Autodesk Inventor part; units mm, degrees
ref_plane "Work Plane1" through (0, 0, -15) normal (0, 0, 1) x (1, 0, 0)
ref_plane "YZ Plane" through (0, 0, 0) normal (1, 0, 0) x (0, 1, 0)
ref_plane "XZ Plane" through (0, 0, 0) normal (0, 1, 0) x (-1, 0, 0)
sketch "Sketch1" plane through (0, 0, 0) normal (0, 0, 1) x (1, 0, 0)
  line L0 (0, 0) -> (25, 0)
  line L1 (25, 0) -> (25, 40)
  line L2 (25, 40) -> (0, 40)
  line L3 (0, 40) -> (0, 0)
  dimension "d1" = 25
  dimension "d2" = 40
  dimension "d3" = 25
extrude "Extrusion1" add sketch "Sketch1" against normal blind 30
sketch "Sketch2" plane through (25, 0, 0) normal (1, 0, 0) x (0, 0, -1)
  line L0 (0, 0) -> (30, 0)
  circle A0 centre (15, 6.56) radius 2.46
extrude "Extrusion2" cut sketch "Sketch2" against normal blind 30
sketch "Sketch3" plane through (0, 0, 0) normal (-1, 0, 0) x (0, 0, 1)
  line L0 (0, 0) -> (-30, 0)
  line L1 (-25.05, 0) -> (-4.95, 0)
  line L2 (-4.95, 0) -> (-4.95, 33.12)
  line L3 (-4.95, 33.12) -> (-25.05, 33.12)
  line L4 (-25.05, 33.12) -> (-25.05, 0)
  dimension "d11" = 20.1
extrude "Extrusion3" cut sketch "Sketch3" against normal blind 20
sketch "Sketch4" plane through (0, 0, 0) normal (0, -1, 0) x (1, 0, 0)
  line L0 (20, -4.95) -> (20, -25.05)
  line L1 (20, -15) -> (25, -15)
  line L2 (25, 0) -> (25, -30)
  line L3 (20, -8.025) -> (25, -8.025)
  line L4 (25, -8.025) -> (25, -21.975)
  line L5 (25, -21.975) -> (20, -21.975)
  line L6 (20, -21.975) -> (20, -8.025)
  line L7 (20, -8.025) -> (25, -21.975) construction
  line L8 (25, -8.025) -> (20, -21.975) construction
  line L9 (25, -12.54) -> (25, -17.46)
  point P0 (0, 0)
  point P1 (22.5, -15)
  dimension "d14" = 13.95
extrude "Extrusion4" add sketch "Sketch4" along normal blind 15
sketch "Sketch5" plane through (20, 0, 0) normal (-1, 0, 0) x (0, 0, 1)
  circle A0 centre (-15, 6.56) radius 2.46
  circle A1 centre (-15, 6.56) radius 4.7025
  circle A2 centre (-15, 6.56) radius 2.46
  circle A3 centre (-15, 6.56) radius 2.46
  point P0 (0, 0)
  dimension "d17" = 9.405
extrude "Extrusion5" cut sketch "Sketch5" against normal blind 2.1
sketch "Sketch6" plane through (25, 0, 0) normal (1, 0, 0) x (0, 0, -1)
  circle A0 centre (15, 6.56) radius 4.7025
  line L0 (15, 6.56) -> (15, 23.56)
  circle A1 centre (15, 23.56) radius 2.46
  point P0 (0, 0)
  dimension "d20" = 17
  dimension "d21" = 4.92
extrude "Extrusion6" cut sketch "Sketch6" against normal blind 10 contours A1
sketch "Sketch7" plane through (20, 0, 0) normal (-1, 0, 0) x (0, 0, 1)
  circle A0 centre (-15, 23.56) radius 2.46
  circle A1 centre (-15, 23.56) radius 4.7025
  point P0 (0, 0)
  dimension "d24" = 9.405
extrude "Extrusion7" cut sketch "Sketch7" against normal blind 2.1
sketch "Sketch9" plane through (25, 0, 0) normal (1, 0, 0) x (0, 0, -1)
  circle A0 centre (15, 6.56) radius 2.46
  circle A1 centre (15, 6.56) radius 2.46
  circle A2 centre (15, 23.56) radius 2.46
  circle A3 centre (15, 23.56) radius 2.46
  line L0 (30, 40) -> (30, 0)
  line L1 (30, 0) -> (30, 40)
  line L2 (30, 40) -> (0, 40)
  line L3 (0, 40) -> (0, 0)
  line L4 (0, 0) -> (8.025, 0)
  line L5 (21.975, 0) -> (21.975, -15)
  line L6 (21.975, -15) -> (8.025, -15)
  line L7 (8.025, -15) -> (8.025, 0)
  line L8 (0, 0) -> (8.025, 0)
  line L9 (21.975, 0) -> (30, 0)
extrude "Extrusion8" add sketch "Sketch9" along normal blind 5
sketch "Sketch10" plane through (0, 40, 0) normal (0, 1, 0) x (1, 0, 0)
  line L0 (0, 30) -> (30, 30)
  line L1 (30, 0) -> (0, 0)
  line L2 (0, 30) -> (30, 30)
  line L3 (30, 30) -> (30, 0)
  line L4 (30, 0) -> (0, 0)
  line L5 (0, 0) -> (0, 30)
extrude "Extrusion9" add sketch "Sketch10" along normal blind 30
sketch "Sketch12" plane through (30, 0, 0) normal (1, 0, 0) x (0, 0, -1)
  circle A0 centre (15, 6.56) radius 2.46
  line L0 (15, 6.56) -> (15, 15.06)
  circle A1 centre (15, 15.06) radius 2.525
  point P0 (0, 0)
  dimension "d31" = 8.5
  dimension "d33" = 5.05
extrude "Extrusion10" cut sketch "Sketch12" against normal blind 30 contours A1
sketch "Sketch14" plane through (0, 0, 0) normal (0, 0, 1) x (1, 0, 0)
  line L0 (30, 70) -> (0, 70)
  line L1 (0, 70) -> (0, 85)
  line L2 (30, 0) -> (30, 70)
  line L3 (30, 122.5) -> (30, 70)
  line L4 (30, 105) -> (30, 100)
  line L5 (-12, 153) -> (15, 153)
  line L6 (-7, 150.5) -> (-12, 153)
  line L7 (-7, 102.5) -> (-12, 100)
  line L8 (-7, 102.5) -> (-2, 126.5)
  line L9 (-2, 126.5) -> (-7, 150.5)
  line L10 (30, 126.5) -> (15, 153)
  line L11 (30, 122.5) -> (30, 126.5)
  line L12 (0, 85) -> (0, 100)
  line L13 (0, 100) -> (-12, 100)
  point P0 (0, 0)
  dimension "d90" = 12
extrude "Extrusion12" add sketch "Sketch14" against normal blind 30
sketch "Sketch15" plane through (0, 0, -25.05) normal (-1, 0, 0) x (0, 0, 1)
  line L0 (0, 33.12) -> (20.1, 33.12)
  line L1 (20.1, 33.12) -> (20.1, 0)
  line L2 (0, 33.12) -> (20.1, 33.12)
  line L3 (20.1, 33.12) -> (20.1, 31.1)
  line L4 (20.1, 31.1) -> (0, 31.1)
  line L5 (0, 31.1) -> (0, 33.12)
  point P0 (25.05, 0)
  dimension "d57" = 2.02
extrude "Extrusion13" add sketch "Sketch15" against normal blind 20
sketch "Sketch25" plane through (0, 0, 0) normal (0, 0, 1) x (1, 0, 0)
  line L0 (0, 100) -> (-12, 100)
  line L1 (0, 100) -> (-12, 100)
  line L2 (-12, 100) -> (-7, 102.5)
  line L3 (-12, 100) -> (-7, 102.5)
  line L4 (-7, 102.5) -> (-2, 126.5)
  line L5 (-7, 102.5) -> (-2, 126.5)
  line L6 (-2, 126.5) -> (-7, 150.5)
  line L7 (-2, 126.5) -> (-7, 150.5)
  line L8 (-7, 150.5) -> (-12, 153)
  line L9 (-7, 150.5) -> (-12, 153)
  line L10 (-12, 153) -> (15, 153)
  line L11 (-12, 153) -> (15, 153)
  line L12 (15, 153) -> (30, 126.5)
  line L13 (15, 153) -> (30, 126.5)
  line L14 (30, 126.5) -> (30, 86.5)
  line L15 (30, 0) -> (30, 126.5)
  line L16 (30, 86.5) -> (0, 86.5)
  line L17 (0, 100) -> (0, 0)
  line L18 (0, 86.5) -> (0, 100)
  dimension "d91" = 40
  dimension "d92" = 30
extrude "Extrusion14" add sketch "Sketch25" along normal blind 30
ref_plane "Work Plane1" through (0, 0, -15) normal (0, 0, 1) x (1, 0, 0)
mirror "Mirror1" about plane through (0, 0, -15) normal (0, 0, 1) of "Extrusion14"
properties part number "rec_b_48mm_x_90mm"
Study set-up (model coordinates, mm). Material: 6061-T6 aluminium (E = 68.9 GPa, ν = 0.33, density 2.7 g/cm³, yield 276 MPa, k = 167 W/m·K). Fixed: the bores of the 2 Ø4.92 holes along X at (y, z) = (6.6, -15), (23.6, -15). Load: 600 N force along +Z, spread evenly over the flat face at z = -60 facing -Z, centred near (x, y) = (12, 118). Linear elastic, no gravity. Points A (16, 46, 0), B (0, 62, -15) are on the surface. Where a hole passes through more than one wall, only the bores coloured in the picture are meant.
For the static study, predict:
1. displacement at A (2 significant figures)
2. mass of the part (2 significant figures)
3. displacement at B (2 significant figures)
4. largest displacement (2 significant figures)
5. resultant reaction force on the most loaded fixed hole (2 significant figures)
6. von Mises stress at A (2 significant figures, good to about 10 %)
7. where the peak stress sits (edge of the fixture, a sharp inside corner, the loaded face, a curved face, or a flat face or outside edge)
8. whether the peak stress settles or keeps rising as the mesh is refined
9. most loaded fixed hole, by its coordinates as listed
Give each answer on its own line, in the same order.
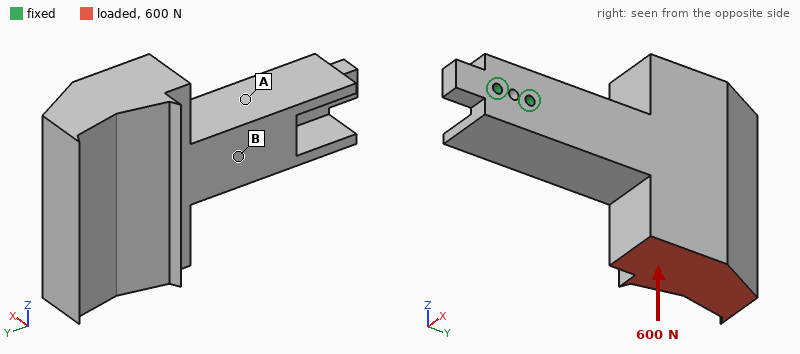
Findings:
0.027 mm
680 g
0.040 mm
0.17 mm
3.0 kN
10 MPa
edge of the fixture
keeps rising
(23.6, -15)
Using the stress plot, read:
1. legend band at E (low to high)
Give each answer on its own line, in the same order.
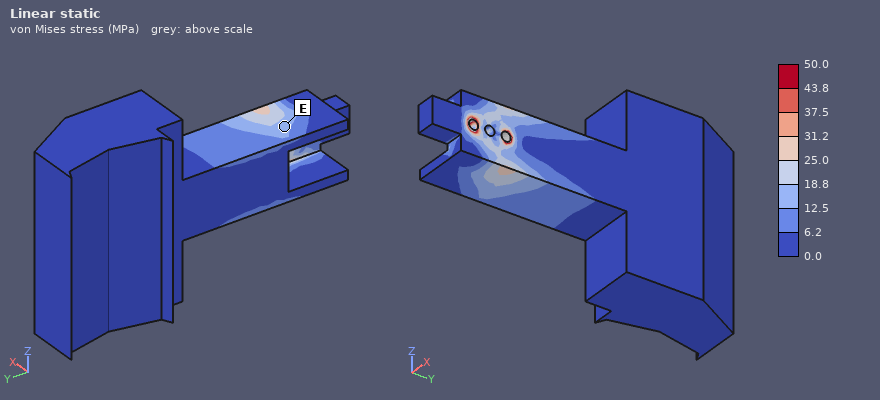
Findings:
12.5 to 18.8 MPa
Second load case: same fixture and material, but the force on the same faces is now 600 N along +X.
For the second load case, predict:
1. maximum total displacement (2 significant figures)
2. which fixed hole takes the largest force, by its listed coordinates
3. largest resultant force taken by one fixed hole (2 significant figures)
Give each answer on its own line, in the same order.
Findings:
0.31 mm
(23.6, -15)
2.9 kN
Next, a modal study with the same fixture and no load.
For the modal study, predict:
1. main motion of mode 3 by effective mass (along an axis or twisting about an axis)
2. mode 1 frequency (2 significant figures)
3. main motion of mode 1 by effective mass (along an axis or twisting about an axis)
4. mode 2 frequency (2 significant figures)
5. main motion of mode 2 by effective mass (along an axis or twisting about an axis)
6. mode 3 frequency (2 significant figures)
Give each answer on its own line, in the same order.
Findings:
twisting about Y
430 Hz
along X
480 Hz
along Z
960 Hz
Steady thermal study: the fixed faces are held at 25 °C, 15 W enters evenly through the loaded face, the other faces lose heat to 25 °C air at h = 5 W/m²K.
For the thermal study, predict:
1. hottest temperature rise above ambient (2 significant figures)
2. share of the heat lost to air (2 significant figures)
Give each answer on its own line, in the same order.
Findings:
11 K
8.2 %
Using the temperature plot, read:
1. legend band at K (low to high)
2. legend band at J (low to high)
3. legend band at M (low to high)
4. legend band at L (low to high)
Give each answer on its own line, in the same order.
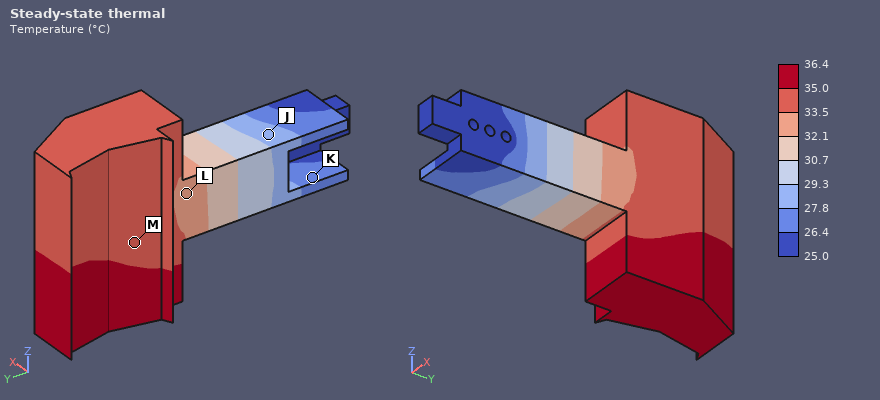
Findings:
26.4 to 27.8 °C
27.8 to 29.3 °C
33.5 to 35.0 °C
32.1 to 33.5 °C
